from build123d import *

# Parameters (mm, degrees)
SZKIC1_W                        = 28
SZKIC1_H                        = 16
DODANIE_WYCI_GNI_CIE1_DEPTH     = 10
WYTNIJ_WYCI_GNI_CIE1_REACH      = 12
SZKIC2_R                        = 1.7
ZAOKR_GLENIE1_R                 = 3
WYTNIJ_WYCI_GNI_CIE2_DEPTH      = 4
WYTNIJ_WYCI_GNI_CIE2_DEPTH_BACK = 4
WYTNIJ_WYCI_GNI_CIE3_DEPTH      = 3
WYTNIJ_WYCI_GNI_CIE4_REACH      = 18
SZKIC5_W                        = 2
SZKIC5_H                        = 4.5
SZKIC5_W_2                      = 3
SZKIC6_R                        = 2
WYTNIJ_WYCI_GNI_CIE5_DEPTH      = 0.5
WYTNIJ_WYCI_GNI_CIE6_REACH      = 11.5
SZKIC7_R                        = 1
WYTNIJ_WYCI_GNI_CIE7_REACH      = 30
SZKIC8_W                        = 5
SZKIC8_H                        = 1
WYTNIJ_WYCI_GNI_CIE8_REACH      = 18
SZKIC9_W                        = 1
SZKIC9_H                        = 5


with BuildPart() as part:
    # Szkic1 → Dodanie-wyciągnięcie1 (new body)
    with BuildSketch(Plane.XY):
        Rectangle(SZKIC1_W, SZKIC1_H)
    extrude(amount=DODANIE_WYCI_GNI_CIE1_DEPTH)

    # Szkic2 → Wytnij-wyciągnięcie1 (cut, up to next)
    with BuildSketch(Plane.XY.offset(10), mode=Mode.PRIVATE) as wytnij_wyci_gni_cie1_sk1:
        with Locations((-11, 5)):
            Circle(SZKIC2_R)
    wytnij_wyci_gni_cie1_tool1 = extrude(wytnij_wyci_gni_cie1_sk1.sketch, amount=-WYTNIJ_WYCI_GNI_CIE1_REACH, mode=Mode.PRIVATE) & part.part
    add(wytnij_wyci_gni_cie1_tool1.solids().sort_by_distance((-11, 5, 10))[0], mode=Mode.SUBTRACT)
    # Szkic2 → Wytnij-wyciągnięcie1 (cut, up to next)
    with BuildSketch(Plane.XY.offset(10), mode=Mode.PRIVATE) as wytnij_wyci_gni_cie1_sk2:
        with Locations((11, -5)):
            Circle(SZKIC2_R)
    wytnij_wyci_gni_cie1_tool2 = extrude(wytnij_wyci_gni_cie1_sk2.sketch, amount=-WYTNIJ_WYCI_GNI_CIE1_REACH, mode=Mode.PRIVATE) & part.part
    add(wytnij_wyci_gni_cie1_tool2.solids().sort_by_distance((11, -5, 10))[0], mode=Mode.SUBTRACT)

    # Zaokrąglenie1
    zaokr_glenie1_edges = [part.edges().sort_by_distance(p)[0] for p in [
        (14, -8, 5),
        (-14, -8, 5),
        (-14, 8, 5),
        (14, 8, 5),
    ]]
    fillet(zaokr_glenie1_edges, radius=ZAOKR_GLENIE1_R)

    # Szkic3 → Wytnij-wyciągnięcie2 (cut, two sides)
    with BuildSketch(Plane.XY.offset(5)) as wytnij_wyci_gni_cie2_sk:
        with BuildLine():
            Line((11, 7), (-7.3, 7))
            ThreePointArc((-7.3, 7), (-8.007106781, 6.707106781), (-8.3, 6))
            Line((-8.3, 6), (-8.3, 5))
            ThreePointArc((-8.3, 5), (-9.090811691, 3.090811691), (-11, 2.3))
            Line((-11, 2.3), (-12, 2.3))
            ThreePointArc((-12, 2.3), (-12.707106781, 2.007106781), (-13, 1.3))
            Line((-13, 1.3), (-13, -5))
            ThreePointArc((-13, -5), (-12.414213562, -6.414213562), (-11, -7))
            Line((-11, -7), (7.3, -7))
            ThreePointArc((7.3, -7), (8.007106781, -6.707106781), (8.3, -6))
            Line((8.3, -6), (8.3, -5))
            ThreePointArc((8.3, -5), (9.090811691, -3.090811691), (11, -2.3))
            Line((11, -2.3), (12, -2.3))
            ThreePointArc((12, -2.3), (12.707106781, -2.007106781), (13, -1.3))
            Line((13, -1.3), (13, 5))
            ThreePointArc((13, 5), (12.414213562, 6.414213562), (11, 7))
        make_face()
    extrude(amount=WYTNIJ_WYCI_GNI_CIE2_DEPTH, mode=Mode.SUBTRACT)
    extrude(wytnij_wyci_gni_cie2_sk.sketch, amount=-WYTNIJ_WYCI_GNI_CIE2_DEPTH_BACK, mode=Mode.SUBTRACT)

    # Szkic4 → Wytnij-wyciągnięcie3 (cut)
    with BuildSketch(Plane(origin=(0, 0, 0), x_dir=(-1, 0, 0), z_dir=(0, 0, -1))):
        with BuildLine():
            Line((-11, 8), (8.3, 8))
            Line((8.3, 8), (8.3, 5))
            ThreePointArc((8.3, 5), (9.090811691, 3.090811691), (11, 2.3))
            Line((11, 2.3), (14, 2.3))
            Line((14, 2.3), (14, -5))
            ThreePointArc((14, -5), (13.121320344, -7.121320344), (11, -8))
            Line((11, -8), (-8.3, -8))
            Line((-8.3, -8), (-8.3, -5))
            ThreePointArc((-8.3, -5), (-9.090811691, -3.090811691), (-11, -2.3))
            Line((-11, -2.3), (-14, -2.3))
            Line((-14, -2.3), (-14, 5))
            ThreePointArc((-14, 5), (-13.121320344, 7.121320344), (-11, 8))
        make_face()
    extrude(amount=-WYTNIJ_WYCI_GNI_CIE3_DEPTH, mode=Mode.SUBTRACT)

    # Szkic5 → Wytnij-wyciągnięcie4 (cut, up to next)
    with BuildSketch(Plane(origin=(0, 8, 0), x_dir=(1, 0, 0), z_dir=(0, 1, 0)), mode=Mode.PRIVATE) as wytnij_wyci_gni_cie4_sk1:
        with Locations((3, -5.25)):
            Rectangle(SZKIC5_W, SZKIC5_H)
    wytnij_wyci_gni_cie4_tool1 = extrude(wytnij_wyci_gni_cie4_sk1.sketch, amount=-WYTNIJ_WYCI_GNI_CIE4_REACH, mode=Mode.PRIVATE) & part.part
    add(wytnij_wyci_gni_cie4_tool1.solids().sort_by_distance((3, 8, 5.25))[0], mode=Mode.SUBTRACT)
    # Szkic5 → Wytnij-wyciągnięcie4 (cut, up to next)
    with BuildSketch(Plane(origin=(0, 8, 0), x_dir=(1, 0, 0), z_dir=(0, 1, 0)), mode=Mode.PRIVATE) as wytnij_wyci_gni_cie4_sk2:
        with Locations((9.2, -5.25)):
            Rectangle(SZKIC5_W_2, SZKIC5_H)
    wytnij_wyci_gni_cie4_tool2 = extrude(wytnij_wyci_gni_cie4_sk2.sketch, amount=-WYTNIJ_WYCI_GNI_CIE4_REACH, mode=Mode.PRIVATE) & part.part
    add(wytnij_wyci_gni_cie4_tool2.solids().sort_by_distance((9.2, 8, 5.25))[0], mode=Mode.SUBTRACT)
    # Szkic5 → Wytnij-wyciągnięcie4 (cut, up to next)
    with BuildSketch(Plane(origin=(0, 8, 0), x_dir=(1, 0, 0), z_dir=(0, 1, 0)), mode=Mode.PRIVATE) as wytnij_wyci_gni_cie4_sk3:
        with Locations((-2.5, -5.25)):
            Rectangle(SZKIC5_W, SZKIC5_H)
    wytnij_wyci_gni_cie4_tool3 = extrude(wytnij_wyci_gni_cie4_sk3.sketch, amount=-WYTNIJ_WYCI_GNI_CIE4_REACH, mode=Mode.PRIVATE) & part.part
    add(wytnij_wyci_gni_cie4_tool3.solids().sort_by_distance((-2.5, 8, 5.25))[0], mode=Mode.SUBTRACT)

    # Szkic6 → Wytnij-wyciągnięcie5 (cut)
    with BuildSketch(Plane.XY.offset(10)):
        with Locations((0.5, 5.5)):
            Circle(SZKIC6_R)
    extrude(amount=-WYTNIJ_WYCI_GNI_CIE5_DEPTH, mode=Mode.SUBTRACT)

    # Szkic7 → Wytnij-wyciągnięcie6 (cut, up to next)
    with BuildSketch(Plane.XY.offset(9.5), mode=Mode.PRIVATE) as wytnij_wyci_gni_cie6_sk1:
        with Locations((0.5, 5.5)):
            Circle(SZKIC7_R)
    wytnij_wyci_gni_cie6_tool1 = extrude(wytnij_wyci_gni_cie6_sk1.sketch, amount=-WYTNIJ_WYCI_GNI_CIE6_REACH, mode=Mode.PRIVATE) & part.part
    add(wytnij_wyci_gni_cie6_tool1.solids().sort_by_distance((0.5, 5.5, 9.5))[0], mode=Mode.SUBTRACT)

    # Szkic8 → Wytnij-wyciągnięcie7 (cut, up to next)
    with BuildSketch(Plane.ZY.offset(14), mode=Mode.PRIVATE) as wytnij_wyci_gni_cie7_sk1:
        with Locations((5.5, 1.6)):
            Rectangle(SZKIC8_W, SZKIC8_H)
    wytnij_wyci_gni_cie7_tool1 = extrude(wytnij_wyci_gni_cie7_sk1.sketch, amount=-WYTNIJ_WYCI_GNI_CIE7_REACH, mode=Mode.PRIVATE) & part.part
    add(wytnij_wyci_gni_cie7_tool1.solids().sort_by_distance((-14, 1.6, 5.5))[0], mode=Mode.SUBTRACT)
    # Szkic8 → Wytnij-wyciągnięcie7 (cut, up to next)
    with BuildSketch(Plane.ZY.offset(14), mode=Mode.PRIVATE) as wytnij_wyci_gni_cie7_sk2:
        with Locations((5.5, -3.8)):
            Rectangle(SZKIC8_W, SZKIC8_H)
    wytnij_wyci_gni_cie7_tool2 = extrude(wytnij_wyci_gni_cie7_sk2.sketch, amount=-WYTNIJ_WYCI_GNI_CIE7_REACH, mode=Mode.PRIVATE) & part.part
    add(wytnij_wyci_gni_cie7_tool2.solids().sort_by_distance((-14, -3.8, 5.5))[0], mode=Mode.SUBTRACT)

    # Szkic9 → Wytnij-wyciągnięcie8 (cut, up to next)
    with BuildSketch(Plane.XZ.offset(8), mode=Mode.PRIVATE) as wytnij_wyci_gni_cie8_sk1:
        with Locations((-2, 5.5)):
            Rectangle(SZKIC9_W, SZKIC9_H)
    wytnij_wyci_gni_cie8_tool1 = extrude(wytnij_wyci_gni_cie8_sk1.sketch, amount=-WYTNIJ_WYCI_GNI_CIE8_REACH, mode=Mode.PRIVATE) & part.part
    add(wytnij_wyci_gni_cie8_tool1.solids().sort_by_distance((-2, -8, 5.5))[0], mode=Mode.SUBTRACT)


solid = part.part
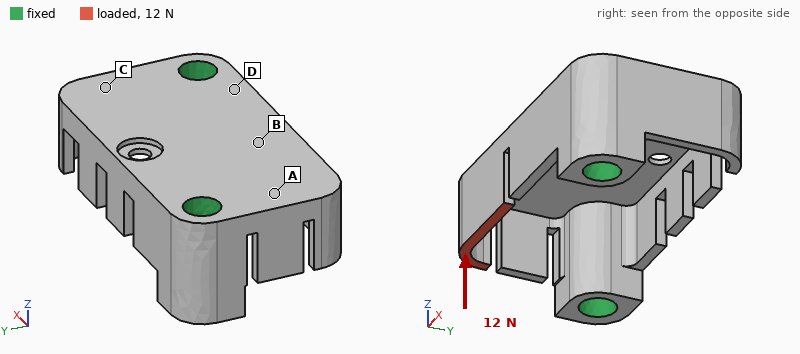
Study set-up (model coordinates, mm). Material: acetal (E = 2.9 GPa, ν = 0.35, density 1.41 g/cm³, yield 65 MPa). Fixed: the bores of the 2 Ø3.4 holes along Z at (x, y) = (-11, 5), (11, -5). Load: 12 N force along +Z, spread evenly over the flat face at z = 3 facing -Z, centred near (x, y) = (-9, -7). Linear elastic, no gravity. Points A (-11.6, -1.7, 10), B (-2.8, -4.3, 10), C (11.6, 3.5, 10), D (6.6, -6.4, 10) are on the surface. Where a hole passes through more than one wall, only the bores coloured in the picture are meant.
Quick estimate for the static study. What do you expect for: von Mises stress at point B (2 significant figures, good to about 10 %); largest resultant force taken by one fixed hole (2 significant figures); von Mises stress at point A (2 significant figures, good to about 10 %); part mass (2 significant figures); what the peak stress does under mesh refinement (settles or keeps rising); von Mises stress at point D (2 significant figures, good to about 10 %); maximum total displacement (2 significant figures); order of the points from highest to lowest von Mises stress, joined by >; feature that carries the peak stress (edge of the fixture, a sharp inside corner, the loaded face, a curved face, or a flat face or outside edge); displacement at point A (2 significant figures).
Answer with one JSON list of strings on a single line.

["5.3 MPa", "11 N", "6.9 MPa", "1.5 g", "keeps rising", "2.6 MPa", "0.35 mm", "A > B > D > C", "a sharp inside corner", "0.074 mm"]
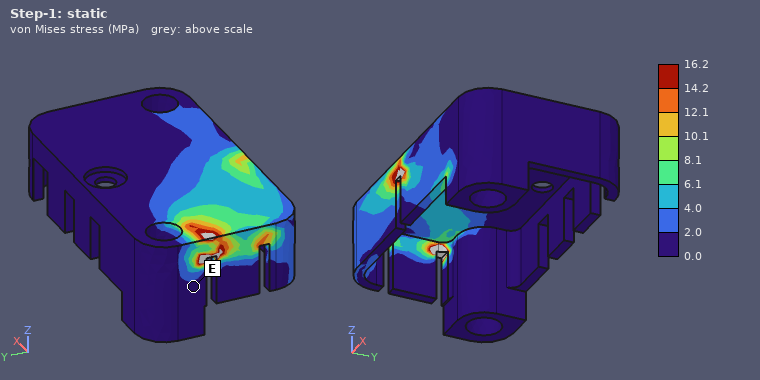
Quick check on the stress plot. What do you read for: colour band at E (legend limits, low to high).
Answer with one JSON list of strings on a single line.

["0.0 to 2.0 MPa"]
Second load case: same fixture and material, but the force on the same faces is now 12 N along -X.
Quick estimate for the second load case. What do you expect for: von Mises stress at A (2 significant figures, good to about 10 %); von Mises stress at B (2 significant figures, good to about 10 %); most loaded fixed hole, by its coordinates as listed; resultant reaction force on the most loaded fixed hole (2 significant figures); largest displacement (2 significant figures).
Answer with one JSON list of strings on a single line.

["6.5 MPa", "4.9 MPa", "(11, -5)", "12 N", "0.34 mm"]
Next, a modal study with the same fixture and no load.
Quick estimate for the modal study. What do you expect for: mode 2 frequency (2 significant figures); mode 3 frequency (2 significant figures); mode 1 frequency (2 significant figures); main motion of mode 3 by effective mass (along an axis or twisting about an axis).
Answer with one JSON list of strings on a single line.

["4200 Hz", "4400 Hz", "2600 Hz", "along Z"]
